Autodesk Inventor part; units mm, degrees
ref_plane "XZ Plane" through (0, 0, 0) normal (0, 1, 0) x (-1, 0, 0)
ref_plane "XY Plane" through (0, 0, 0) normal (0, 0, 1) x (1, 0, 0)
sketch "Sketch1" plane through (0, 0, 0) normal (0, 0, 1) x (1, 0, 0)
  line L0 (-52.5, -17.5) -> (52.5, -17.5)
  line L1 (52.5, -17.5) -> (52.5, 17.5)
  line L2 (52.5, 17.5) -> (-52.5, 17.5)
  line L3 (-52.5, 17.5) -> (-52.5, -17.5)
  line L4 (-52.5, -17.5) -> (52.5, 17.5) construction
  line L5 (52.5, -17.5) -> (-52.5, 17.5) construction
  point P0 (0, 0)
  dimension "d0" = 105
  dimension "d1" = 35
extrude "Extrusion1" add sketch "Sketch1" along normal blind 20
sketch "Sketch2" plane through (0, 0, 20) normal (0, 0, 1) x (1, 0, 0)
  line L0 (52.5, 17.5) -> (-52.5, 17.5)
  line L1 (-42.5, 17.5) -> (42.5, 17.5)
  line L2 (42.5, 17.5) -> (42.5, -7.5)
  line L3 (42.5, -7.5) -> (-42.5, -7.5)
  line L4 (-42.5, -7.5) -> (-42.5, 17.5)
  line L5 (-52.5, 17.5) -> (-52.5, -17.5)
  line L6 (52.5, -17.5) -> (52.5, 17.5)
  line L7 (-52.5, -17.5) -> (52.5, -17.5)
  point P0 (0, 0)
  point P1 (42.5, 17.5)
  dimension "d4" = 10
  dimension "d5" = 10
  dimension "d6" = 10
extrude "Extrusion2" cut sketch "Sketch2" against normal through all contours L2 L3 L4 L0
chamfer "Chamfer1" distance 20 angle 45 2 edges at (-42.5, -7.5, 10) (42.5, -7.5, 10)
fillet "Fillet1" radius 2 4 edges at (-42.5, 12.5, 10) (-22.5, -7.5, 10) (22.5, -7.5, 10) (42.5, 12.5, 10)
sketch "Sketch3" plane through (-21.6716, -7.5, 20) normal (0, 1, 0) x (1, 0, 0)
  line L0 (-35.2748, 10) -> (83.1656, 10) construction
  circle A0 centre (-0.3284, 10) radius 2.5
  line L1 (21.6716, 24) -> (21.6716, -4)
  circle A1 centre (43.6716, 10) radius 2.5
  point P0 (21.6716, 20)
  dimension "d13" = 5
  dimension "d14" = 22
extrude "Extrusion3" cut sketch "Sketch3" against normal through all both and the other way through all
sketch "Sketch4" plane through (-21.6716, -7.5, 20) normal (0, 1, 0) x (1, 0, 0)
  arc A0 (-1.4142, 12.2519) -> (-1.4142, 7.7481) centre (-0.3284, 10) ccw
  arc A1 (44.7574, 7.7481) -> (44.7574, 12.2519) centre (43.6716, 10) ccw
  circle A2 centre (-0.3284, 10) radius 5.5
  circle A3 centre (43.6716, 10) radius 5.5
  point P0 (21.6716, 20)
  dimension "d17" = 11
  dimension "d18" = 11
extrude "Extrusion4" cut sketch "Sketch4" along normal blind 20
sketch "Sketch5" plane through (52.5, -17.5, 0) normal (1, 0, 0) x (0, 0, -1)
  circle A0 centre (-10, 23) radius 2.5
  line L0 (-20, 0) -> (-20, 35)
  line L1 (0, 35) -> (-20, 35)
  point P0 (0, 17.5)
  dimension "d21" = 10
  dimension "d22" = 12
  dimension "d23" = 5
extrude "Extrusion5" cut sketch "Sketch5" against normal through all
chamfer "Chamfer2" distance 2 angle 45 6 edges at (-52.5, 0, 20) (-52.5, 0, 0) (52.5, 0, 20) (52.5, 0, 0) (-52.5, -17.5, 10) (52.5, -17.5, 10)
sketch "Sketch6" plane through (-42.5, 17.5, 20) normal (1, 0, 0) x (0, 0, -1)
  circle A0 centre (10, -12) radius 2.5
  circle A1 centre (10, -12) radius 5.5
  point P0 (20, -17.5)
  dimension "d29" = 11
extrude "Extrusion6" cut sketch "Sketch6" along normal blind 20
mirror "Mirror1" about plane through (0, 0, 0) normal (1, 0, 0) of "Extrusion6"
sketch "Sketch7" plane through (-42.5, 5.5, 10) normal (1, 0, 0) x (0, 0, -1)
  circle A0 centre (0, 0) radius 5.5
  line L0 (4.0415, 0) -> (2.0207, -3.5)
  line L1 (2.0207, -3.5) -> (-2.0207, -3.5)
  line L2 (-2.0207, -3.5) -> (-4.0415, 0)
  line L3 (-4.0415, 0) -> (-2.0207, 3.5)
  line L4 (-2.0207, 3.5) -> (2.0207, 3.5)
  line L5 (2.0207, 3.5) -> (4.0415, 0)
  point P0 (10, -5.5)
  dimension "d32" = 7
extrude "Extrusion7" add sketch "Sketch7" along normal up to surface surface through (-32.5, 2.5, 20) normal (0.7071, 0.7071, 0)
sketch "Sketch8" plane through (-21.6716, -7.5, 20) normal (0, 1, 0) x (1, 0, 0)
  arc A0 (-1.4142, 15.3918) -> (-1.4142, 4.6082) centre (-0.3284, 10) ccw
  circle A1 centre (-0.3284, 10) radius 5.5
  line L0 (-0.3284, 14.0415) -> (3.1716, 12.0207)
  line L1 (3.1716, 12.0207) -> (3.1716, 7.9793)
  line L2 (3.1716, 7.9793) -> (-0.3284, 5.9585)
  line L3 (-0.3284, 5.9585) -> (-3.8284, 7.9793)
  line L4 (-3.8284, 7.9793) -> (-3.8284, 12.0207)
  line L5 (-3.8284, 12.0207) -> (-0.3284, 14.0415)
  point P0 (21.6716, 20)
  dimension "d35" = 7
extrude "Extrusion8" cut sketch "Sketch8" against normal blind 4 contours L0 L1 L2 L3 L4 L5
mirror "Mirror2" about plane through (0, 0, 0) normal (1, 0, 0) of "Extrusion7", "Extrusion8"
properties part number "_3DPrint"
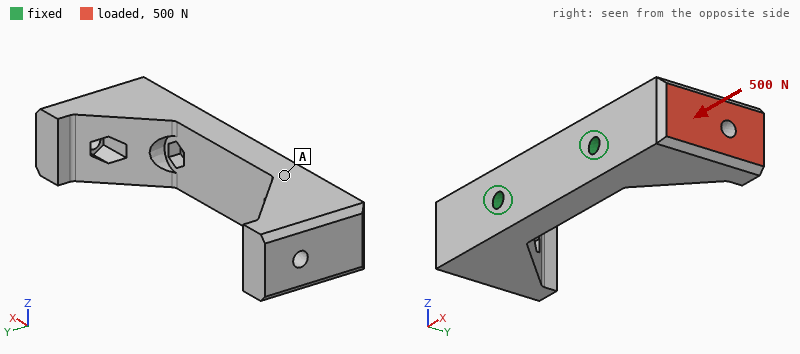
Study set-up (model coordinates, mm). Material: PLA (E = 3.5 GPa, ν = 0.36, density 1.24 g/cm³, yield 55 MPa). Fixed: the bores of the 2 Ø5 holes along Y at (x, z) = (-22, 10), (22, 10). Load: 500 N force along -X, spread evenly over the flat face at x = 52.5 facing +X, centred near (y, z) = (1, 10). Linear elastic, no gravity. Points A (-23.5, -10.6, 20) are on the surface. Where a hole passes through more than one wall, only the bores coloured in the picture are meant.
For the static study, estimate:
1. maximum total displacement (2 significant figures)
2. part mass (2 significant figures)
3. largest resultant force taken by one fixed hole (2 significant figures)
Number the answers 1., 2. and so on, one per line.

1. 0.68 mm
2. 46 g
3. 270 N
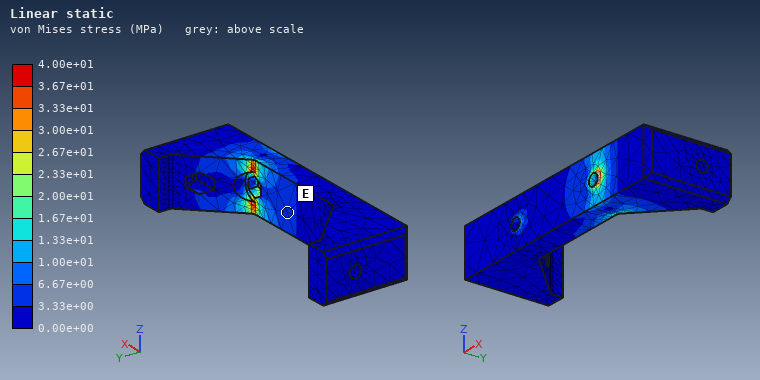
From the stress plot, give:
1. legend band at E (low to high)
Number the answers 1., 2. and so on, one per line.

1. 3.33e+00 to 6.67e+00 MPa
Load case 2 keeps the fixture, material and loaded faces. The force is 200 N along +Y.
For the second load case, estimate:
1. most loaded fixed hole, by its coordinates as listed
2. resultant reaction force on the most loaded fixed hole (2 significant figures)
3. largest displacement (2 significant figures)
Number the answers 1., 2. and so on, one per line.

1. (22, 10)
2. 310 N
3. 0.54 mm
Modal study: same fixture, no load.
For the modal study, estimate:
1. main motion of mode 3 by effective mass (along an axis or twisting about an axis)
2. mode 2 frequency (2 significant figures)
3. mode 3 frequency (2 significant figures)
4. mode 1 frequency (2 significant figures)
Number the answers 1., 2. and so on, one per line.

1. along Z
2. 1200 Hz
3. 1400 Hz
4. 1100 Hz
